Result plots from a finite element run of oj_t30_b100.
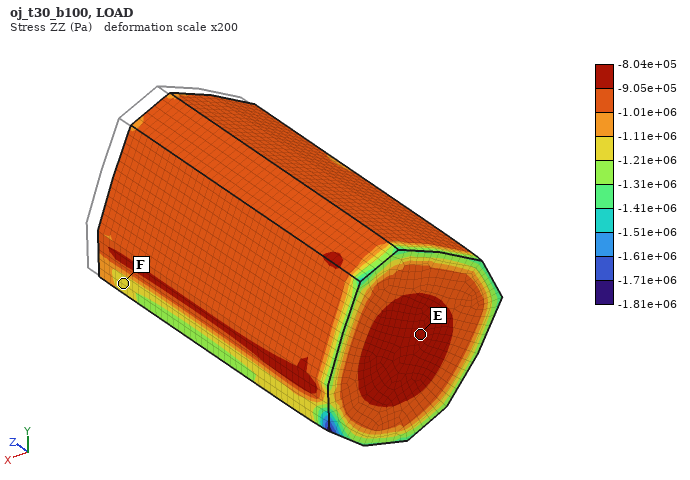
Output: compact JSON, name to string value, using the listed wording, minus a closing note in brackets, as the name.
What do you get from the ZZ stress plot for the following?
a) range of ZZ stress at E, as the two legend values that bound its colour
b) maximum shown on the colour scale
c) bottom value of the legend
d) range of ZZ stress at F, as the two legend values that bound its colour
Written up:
{"range of ZZ stress at E, as the two legend values that bound its colour": "-9.05e+05 to -8.04e+05 Pa", "maximum shown on the colour scale": "-8.04e+05 Pa", "bottom value of the legend": "-1.81e+06 Pa", "range of ZZ stress at F, as the two legend values that bound its colour": "-1.21e+06 to -1.11e+06 Pa"}
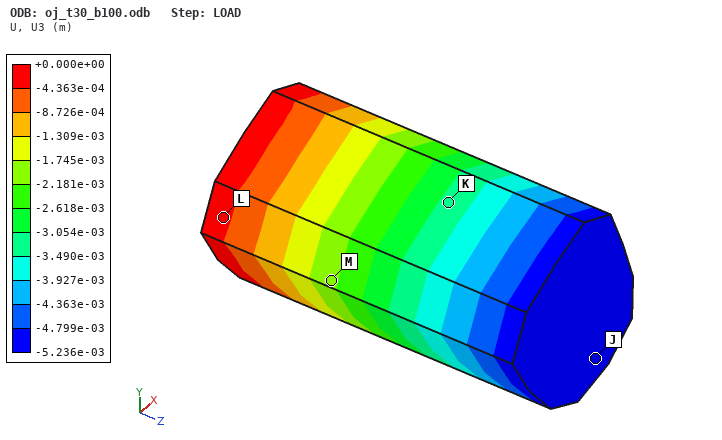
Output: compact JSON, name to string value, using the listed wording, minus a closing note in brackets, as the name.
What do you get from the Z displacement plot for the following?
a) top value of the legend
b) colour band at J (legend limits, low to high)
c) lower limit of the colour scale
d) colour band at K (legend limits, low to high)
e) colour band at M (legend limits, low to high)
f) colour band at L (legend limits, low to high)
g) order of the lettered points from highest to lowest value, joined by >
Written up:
{"top value of the legend": "+0.000e+00 m", "colour band at J": "-5.236e-03 to -4.799e-03 m", "lower limit of the colour scale": "-5.236e-03 m", "colour band at K": "-3.490e-03 to -3.054e-03 m", "colour band at M": "-2.181e-03 to -1.745e-03 m", "colour band at L": "-4.363e-04 to +0.000e+00 m", "order of the lettered points from highest to lowest value, joined by >": "L > M > K > J"}
